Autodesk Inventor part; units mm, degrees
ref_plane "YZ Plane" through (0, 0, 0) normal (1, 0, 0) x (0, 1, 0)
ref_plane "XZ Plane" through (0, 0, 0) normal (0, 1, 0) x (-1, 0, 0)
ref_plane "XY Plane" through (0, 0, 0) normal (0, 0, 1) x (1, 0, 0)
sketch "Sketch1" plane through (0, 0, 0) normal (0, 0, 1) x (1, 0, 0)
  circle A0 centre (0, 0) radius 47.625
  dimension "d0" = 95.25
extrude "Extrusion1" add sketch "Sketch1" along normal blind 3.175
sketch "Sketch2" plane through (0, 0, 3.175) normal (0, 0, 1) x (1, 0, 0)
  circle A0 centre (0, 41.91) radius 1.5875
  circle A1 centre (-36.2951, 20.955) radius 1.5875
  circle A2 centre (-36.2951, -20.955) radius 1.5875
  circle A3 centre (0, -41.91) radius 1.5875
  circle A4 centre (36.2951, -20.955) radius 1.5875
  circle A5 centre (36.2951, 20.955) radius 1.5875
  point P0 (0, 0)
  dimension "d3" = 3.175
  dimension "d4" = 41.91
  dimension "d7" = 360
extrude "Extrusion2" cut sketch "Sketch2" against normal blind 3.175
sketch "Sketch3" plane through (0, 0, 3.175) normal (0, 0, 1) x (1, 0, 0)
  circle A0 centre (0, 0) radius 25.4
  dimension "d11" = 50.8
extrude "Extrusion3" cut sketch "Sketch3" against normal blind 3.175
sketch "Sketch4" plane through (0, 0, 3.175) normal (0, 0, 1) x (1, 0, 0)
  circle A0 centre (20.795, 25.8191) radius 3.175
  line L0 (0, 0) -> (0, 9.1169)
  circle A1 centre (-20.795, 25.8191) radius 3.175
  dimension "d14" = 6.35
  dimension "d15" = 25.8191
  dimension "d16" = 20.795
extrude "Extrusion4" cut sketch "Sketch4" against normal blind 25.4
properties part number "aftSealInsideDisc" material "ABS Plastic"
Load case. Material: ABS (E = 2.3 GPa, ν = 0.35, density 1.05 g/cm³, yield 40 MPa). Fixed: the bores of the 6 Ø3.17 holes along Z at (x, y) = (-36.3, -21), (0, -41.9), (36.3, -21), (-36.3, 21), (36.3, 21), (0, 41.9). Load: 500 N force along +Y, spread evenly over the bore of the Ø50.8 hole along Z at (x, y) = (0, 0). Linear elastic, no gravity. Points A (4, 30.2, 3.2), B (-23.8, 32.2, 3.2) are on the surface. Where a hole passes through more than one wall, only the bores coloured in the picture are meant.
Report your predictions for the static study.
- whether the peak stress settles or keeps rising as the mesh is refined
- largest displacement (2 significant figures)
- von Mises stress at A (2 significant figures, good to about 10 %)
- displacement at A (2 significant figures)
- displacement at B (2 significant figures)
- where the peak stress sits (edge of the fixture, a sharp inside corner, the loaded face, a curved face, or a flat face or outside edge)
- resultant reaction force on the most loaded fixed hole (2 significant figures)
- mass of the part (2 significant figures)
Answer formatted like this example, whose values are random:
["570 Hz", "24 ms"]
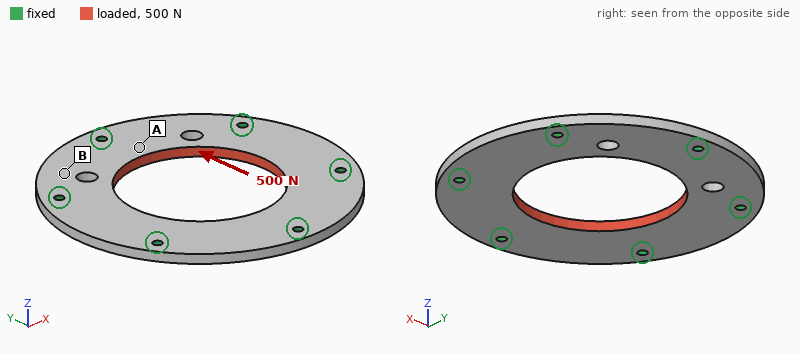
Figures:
["keeps rising", "22 µm", "1.6 MPa", "13 µm", "14 µm", "edge of the fixture", "100 N", "17 g"]
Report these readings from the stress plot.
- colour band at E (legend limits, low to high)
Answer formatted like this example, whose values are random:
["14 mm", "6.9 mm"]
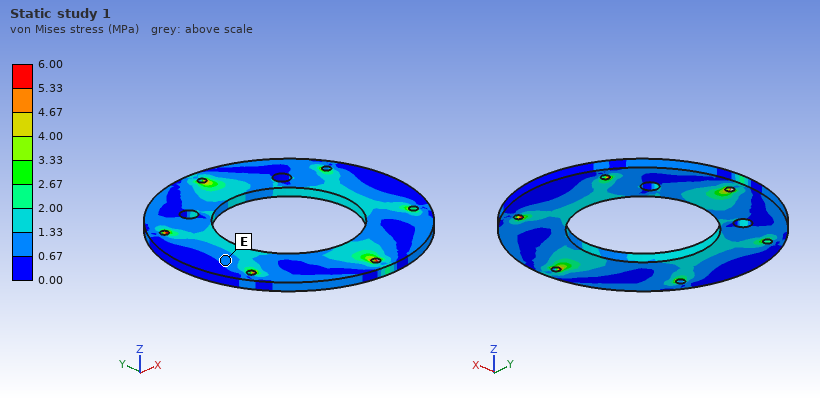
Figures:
["0.67 to 1.33 MPa"]
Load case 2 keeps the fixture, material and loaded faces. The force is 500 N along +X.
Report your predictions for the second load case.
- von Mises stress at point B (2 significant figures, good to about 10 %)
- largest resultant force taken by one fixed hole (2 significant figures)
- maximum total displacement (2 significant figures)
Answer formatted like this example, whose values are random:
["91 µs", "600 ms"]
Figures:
["1.1 MPa", "96 N", "22 µm"]
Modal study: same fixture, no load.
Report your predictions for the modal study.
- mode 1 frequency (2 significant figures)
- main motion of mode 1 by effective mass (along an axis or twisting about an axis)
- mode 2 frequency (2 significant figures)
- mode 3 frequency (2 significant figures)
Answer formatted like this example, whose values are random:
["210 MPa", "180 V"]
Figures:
["2100 Hz", "along Z", "2300 Hz", "2400 Hz"]
